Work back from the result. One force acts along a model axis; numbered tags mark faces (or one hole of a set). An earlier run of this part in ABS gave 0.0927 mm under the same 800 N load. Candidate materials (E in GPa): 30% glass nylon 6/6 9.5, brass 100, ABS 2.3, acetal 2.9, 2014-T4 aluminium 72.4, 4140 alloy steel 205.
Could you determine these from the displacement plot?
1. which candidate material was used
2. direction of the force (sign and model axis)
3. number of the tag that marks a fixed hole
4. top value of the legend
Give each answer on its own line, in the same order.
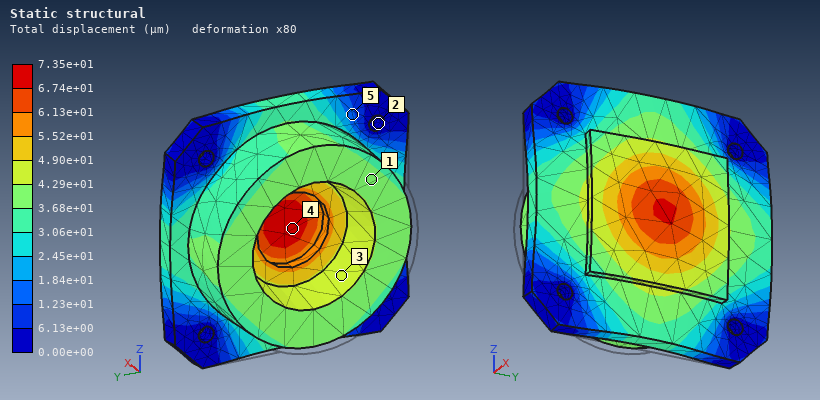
acetal
+X
2
7.35e+01 µm
